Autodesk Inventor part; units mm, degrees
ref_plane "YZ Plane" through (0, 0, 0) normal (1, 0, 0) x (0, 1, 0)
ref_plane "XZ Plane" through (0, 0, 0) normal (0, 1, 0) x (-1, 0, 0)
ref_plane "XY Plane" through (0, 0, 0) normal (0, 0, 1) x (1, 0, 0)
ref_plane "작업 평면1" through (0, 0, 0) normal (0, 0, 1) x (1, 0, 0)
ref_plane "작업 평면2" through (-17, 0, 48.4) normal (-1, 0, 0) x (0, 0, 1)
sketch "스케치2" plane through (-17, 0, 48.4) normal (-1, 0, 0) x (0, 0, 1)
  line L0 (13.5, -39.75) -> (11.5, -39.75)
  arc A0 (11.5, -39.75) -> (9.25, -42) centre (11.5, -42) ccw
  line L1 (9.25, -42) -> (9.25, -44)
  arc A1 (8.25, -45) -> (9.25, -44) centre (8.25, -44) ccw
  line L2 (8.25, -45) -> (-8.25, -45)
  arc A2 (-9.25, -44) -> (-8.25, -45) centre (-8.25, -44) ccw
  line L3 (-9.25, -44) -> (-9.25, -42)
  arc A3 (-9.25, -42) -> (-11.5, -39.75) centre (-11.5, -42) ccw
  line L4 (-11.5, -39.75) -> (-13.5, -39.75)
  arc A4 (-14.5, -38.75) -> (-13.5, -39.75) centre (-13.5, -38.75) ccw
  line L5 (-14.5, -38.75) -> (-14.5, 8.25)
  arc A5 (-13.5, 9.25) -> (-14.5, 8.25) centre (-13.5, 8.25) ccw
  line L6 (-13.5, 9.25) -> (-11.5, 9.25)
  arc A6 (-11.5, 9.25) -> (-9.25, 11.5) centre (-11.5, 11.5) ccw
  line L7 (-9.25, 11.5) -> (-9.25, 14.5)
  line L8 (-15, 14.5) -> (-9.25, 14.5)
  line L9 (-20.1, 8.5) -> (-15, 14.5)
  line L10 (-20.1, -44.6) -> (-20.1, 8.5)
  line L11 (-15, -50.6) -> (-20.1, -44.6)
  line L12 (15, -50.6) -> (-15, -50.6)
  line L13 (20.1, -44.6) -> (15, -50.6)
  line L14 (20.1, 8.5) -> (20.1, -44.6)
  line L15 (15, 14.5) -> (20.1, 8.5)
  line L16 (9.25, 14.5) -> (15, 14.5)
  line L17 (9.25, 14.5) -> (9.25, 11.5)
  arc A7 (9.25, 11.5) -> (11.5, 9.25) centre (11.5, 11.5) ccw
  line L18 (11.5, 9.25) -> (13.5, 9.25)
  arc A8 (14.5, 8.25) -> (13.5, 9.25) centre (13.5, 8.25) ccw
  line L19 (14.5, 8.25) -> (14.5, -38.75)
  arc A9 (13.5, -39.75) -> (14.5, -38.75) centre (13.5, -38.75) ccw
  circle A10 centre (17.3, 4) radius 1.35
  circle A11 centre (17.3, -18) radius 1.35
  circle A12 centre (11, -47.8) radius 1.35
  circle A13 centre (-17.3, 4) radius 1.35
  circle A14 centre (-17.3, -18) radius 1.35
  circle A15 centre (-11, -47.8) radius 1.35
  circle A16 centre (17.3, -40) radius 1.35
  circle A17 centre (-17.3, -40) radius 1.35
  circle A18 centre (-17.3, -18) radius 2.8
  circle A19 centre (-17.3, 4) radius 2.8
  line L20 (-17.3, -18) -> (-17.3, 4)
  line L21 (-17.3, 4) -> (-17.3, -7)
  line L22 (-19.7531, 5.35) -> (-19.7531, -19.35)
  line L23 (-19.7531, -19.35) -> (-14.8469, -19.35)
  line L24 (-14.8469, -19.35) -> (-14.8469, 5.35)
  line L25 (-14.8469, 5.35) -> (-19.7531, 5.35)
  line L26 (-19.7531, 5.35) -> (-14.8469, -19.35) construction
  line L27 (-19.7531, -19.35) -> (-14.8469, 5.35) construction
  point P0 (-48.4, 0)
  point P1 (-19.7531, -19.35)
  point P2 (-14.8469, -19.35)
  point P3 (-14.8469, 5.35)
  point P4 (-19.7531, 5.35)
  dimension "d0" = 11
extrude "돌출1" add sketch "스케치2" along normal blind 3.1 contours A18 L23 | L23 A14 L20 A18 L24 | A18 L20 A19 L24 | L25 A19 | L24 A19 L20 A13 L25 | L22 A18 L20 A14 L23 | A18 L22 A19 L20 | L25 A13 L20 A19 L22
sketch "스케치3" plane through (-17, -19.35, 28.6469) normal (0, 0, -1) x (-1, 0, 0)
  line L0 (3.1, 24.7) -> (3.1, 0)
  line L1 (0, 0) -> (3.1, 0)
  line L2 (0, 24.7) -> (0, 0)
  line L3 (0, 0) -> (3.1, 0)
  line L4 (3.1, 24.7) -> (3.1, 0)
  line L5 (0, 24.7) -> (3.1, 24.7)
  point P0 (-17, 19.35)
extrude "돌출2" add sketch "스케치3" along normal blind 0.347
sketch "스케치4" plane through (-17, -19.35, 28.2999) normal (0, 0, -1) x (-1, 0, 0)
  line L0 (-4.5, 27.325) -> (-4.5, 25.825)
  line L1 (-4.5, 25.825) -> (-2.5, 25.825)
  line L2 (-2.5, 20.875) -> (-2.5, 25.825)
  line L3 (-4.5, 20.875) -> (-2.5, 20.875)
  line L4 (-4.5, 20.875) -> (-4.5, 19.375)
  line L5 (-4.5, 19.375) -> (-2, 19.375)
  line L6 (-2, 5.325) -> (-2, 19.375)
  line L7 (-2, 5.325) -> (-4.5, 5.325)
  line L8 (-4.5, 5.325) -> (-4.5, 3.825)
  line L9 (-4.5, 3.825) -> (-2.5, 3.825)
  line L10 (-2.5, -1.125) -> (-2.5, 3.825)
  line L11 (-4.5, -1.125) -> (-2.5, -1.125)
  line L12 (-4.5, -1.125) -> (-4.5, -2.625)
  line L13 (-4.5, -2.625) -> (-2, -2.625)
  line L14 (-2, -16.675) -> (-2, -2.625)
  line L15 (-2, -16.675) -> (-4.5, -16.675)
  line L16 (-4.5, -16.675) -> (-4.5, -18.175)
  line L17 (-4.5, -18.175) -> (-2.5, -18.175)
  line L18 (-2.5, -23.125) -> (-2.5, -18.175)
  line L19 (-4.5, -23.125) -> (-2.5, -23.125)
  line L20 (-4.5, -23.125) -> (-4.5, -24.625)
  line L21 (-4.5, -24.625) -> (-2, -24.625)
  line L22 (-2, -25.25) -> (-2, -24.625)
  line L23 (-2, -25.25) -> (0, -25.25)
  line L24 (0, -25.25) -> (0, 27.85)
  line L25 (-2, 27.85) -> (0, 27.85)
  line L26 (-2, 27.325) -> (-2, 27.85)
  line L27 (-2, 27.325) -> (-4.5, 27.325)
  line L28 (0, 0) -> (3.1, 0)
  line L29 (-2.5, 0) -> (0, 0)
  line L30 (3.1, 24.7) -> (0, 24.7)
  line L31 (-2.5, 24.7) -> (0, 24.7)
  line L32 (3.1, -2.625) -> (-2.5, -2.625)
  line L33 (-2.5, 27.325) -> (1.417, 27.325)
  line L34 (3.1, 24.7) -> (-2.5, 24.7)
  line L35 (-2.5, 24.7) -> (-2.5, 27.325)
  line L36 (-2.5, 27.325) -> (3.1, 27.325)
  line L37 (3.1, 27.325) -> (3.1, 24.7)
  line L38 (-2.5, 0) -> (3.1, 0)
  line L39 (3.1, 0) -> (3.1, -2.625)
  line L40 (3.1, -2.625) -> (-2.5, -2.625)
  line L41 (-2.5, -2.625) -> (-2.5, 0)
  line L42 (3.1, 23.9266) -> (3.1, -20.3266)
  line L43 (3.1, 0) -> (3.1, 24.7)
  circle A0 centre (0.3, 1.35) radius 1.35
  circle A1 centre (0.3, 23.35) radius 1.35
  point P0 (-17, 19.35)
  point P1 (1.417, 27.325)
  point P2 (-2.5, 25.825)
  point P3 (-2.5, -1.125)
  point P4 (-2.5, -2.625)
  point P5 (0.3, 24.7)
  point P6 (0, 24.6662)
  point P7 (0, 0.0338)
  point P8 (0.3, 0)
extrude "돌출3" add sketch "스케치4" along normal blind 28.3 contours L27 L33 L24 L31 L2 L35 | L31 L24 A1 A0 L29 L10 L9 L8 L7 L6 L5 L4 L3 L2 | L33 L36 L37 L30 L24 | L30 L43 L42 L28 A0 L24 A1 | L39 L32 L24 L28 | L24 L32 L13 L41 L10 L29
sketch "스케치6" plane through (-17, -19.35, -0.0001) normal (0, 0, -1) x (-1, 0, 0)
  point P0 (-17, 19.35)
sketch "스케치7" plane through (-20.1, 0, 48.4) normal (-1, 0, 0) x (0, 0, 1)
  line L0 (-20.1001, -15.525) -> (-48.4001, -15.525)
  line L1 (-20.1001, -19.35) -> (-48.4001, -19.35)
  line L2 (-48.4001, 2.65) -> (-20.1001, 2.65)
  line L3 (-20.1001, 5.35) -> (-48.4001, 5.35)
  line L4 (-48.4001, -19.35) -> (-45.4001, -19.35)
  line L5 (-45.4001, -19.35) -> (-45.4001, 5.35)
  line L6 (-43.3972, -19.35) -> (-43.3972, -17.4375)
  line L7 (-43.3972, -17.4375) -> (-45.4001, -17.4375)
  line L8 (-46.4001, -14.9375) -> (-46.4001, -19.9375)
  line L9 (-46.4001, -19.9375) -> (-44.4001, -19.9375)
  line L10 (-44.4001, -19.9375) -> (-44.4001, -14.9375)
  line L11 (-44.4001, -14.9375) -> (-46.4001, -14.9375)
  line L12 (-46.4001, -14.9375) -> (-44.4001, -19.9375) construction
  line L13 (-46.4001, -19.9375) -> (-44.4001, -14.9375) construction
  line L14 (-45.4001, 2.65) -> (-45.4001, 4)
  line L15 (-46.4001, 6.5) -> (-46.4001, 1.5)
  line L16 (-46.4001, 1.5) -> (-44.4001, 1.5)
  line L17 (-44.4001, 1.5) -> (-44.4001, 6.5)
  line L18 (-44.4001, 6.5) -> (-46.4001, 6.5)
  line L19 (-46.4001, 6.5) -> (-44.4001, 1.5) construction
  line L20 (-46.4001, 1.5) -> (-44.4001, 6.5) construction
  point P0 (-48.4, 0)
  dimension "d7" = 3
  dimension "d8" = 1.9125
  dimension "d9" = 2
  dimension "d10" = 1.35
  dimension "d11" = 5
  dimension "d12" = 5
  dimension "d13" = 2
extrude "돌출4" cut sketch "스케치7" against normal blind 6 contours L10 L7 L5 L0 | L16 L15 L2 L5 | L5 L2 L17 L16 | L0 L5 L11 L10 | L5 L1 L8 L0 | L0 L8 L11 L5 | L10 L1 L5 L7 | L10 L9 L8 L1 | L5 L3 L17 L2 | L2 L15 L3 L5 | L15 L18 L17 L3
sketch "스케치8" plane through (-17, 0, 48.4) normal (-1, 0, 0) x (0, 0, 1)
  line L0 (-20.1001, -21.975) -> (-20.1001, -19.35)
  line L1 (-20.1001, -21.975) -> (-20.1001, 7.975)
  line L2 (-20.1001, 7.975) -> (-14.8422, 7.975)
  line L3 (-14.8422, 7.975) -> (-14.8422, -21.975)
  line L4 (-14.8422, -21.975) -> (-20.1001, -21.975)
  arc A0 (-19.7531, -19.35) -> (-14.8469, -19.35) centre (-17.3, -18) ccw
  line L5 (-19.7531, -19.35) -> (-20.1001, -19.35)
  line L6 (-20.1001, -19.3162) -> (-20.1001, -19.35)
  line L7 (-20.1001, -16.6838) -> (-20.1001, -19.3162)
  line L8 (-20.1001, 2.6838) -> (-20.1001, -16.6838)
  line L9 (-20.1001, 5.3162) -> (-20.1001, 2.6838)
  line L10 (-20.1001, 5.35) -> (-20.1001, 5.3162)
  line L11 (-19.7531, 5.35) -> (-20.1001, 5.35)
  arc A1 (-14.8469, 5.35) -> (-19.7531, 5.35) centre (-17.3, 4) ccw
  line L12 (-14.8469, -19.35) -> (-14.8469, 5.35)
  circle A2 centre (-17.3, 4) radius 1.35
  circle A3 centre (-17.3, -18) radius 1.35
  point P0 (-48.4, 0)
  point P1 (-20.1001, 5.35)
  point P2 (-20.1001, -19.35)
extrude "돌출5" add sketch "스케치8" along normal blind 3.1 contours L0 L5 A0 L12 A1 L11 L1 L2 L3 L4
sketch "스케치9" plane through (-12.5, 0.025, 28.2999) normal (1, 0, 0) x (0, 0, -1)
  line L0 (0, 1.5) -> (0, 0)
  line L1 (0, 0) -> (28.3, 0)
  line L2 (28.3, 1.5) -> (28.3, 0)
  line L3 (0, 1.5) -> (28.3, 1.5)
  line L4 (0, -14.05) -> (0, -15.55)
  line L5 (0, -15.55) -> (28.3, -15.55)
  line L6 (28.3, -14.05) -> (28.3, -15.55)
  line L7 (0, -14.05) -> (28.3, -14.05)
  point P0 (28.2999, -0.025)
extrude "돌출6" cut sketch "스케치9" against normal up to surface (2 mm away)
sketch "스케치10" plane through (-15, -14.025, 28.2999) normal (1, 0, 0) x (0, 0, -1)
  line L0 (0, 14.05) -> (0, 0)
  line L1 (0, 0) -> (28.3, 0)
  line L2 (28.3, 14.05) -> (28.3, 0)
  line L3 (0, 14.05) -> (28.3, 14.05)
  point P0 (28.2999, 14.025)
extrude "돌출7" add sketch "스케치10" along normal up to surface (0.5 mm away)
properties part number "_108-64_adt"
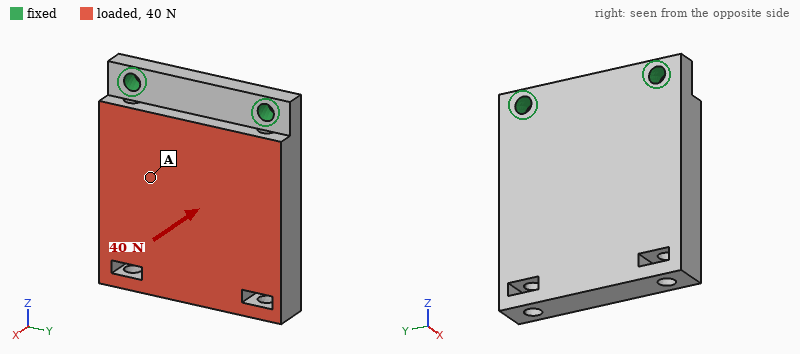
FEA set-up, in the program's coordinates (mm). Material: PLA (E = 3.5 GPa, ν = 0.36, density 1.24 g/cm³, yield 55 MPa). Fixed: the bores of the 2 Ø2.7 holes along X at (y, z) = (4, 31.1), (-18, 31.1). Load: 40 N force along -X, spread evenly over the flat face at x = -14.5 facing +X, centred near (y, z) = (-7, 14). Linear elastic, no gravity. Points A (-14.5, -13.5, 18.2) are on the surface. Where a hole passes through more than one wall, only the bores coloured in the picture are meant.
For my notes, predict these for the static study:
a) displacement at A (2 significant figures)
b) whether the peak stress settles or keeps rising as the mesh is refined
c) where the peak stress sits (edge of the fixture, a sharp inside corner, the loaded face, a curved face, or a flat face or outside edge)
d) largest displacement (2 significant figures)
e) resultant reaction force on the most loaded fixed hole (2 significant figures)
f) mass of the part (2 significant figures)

0.19 mm
keeps rising
a sharp inside corner
0.49 mm
20 N
5.9 g
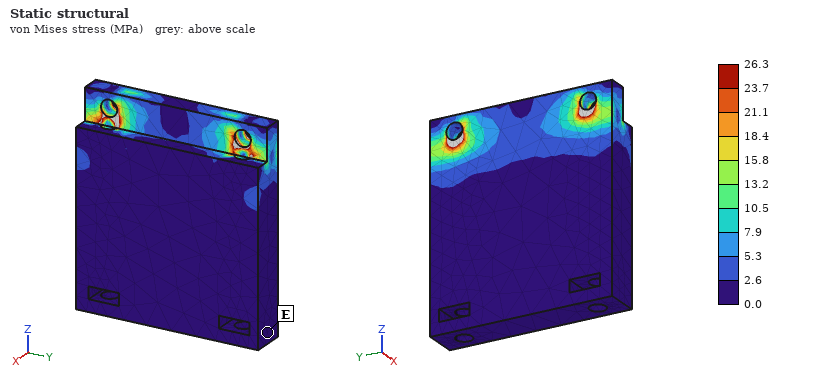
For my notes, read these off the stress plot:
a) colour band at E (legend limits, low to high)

0.0 to 2.6 MPa
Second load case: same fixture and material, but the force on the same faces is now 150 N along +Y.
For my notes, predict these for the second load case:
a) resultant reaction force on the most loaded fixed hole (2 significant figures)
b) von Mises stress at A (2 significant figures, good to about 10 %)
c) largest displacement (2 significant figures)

130 N
2.5 MPa
67 µm
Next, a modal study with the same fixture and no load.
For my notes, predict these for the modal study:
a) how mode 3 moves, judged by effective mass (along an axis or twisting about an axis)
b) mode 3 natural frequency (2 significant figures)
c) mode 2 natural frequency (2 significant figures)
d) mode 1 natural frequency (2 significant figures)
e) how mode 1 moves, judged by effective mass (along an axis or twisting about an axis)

along Y
4500 Hz
3100 Hz
770 Hz
along X
